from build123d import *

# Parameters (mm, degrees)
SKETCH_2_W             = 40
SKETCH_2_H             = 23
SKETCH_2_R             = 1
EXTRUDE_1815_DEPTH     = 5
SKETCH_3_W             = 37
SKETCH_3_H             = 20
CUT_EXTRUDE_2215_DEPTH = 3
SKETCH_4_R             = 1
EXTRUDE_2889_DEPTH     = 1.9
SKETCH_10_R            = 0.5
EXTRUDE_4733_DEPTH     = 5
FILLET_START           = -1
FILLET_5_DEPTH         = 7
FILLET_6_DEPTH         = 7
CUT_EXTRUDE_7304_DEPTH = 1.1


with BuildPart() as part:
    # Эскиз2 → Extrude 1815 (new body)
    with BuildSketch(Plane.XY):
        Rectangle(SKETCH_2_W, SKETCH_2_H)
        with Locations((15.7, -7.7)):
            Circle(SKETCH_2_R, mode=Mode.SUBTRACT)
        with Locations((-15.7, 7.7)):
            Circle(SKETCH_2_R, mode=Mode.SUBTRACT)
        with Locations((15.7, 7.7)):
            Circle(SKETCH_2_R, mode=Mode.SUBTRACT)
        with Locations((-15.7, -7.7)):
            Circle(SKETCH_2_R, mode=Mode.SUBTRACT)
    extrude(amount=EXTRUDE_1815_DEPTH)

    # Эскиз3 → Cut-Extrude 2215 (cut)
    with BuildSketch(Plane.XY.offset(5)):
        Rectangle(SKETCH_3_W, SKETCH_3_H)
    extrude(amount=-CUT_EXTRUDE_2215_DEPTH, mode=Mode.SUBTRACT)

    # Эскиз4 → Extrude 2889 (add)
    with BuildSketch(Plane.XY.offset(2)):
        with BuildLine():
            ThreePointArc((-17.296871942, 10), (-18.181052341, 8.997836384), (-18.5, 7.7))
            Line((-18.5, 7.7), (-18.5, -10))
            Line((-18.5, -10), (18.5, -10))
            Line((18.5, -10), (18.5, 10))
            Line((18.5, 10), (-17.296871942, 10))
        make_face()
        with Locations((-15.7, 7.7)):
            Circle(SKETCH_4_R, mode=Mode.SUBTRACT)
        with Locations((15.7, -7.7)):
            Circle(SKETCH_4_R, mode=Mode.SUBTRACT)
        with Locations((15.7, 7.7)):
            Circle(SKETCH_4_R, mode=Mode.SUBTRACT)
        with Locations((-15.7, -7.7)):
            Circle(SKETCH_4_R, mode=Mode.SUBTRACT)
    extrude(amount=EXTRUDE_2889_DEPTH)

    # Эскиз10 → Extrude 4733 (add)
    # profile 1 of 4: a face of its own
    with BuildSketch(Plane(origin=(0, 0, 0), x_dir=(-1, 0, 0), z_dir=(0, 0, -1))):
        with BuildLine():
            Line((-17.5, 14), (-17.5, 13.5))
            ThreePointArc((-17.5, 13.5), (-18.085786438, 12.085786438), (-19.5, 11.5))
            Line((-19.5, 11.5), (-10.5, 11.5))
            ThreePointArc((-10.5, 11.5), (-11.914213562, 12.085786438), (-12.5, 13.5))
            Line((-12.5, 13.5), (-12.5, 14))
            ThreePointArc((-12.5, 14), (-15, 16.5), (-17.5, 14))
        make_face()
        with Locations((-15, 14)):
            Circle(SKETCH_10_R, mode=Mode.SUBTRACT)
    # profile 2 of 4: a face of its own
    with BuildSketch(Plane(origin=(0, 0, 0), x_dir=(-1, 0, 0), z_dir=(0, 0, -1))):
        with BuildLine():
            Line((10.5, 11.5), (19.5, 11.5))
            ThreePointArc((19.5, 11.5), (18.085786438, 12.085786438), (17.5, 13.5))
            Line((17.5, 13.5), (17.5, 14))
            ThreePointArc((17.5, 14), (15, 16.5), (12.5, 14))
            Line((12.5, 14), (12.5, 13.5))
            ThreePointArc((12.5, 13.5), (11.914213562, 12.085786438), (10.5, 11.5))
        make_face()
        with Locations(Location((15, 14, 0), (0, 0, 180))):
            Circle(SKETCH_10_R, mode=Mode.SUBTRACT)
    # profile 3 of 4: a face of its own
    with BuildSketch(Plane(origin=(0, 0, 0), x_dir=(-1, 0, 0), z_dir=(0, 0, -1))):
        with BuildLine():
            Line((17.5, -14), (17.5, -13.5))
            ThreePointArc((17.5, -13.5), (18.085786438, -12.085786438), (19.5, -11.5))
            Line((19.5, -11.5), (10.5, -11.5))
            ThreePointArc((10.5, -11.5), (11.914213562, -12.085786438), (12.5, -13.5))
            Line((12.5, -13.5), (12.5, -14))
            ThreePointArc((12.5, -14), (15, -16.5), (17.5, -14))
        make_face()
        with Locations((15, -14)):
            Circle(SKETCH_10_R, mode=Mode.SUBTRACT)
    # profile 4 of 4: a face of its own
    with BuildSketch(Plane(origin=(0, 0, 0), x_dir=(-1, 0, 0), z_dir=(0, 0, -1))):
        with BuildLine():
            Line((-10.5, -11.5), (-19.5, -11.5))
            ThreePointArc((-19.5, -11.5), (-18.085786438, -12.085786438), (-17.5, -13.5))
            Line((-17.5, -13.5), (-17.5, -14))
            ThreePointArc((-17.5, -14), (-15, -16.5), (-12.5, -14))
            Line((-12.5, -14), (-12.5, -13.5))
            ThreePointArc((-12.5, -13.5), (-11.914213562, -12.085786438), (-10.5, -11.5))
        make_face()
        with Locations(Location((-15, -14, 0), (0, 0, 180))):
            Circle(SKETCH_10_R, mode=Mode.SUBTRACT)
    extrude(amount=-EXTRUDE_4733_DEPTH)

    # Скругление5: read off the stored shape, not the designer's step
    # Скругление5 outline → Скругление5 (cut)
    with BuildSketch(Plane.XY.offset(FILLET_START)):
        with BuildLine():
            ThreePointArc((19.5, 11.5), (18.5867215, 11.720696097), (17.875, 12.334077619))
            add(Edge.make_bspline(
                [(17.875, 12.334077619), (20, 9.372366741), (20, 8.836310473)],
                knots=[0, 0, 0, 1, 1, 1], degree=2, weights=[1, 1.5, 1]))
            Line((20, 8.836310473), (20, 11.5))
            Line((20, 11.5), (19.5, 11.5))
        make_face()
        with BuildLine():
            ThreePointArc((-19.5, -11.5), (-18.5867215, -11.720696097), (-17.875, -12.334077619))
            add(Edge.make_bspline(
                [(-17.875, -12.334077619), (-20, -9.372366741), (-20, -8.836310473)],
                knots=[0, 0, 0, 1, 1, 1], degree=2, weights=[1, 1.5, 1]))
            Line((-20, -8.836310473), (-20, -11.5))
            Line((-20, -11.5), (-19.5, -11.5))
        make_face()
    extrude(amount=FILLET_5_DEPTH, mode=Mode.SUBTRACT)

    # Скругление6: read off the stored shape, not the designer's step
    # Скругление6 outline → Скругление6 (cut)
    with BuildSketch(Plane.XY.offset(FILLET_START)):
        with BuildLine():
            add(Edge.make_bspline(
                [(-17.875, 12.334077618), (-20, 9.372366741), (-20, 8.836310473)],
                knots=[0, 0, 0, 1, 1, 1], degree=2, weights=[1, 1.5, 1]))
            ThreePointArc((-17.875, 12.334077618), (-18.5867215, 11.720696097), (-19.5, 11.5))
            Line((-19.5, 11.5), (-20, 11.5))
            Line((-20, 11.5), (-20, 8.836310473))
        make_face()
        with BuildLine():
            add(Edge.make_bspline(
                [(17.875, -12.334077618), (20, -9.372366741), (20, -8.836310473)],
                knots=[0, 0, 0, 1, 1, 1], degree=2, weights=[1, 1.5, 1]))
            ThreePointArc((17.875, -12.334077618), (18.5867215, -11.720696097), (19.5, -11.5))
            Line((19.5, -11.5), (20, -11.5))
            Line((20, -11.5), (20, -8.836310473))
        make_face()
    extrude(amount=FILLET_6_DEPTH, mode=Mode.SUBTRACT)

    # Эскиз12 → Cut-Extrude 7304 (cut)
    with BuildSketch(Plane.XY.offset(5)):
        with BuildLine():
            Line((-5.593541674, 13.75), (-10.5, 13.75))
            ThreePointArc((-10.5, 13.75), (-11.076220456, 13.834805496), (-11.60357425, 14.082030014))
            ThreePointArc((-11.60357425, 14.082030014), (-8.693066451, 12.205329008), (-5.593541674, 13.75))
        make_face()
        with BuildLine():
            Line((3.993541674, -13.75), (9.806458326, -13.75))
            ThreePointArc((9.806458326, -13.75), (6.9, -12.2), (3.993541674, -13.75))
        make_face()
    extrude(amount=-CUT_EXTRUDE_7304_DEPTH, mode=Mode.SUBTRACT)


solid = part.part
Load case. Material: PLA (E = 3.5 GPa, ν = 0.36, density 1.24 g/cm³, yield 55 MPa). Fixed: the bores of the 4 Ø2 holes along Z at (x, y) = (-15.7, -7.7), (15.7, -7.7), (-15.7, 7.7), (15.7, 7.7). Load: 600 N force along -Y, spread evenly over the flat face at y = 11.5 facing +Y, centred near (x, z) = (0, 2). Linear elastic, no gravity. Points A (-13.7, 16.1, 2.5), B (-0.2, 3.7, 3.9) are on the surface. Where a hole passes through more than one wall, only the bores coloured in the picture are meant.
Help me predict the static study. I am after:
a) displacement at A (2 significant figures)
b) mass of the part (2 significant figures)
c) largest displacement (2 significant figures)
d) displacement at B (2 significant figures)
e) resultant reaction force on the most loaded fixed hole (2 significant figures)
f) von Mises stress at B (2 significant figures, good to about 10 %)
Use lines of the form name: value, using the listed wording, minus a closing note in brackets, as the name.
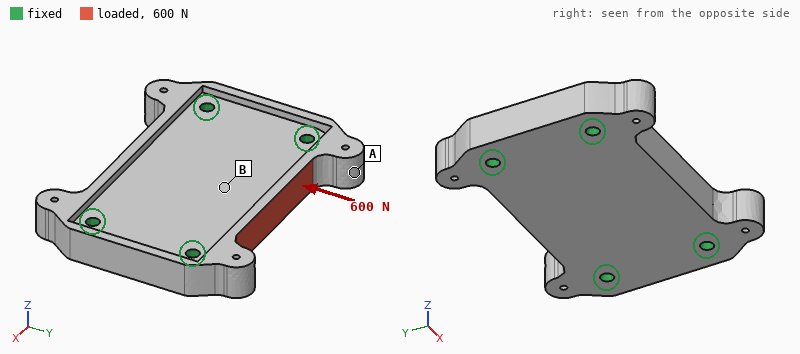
displacement at A: 29 µm
mass of the part: 5.2 g
largest displacement: 90 µm
displacement at B: 45 µm
resultant reaction force on the most loaded fixed hole: 180 N
von Mises stress at B: 7.8 MPa
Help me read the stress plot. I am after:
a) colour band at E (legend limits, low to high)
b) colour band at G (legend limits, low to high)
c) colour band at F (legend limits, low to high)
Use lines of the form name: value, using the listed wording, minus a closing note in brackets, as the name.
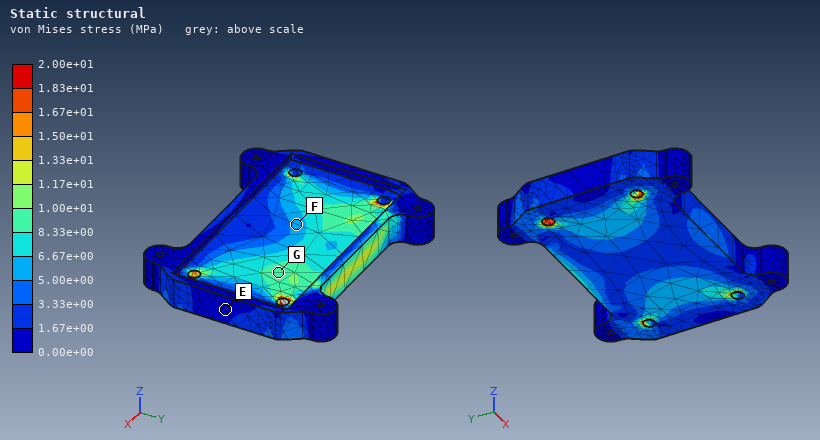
colour band at E: 0.00e+00 to 1.67e+00 MPa
colour band at G: 8.33e+00 to 1.00e+01 MPa
colour band at F: 5.00e+00 to 6.67e+00 MPa
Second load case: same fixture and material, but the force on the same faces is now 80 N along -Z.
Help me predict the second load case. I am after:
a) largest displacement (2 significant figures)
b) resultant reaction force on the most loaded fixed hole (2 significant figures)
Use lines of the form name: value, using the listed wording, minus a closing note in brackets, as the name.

largest displacement: 90 µm
resultant reaction force on the most loaded fixed hole: 46 N
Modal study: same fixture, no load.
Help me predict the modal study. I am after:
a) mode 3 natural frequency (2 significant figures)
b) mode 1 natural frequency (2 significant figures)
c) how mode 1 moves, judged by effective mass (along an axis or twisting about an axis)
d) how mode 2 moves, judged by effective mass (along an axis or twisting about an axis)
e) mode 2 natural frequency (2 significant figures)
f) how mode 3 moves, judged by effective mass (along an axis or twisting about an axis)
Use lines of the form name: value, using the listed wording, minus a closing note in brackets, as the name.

mode 3 natural frequency: 13 kHz
mode 1 natural frequency: 5900 Hz
how mode 1 moves, judged by effective mass: along Z
how mode 2 moves, judged by effective mass: twisting about X
mode 2 natural frequency: 7900 Hz
how mode 3 moves, judged by effective mass: along Y
